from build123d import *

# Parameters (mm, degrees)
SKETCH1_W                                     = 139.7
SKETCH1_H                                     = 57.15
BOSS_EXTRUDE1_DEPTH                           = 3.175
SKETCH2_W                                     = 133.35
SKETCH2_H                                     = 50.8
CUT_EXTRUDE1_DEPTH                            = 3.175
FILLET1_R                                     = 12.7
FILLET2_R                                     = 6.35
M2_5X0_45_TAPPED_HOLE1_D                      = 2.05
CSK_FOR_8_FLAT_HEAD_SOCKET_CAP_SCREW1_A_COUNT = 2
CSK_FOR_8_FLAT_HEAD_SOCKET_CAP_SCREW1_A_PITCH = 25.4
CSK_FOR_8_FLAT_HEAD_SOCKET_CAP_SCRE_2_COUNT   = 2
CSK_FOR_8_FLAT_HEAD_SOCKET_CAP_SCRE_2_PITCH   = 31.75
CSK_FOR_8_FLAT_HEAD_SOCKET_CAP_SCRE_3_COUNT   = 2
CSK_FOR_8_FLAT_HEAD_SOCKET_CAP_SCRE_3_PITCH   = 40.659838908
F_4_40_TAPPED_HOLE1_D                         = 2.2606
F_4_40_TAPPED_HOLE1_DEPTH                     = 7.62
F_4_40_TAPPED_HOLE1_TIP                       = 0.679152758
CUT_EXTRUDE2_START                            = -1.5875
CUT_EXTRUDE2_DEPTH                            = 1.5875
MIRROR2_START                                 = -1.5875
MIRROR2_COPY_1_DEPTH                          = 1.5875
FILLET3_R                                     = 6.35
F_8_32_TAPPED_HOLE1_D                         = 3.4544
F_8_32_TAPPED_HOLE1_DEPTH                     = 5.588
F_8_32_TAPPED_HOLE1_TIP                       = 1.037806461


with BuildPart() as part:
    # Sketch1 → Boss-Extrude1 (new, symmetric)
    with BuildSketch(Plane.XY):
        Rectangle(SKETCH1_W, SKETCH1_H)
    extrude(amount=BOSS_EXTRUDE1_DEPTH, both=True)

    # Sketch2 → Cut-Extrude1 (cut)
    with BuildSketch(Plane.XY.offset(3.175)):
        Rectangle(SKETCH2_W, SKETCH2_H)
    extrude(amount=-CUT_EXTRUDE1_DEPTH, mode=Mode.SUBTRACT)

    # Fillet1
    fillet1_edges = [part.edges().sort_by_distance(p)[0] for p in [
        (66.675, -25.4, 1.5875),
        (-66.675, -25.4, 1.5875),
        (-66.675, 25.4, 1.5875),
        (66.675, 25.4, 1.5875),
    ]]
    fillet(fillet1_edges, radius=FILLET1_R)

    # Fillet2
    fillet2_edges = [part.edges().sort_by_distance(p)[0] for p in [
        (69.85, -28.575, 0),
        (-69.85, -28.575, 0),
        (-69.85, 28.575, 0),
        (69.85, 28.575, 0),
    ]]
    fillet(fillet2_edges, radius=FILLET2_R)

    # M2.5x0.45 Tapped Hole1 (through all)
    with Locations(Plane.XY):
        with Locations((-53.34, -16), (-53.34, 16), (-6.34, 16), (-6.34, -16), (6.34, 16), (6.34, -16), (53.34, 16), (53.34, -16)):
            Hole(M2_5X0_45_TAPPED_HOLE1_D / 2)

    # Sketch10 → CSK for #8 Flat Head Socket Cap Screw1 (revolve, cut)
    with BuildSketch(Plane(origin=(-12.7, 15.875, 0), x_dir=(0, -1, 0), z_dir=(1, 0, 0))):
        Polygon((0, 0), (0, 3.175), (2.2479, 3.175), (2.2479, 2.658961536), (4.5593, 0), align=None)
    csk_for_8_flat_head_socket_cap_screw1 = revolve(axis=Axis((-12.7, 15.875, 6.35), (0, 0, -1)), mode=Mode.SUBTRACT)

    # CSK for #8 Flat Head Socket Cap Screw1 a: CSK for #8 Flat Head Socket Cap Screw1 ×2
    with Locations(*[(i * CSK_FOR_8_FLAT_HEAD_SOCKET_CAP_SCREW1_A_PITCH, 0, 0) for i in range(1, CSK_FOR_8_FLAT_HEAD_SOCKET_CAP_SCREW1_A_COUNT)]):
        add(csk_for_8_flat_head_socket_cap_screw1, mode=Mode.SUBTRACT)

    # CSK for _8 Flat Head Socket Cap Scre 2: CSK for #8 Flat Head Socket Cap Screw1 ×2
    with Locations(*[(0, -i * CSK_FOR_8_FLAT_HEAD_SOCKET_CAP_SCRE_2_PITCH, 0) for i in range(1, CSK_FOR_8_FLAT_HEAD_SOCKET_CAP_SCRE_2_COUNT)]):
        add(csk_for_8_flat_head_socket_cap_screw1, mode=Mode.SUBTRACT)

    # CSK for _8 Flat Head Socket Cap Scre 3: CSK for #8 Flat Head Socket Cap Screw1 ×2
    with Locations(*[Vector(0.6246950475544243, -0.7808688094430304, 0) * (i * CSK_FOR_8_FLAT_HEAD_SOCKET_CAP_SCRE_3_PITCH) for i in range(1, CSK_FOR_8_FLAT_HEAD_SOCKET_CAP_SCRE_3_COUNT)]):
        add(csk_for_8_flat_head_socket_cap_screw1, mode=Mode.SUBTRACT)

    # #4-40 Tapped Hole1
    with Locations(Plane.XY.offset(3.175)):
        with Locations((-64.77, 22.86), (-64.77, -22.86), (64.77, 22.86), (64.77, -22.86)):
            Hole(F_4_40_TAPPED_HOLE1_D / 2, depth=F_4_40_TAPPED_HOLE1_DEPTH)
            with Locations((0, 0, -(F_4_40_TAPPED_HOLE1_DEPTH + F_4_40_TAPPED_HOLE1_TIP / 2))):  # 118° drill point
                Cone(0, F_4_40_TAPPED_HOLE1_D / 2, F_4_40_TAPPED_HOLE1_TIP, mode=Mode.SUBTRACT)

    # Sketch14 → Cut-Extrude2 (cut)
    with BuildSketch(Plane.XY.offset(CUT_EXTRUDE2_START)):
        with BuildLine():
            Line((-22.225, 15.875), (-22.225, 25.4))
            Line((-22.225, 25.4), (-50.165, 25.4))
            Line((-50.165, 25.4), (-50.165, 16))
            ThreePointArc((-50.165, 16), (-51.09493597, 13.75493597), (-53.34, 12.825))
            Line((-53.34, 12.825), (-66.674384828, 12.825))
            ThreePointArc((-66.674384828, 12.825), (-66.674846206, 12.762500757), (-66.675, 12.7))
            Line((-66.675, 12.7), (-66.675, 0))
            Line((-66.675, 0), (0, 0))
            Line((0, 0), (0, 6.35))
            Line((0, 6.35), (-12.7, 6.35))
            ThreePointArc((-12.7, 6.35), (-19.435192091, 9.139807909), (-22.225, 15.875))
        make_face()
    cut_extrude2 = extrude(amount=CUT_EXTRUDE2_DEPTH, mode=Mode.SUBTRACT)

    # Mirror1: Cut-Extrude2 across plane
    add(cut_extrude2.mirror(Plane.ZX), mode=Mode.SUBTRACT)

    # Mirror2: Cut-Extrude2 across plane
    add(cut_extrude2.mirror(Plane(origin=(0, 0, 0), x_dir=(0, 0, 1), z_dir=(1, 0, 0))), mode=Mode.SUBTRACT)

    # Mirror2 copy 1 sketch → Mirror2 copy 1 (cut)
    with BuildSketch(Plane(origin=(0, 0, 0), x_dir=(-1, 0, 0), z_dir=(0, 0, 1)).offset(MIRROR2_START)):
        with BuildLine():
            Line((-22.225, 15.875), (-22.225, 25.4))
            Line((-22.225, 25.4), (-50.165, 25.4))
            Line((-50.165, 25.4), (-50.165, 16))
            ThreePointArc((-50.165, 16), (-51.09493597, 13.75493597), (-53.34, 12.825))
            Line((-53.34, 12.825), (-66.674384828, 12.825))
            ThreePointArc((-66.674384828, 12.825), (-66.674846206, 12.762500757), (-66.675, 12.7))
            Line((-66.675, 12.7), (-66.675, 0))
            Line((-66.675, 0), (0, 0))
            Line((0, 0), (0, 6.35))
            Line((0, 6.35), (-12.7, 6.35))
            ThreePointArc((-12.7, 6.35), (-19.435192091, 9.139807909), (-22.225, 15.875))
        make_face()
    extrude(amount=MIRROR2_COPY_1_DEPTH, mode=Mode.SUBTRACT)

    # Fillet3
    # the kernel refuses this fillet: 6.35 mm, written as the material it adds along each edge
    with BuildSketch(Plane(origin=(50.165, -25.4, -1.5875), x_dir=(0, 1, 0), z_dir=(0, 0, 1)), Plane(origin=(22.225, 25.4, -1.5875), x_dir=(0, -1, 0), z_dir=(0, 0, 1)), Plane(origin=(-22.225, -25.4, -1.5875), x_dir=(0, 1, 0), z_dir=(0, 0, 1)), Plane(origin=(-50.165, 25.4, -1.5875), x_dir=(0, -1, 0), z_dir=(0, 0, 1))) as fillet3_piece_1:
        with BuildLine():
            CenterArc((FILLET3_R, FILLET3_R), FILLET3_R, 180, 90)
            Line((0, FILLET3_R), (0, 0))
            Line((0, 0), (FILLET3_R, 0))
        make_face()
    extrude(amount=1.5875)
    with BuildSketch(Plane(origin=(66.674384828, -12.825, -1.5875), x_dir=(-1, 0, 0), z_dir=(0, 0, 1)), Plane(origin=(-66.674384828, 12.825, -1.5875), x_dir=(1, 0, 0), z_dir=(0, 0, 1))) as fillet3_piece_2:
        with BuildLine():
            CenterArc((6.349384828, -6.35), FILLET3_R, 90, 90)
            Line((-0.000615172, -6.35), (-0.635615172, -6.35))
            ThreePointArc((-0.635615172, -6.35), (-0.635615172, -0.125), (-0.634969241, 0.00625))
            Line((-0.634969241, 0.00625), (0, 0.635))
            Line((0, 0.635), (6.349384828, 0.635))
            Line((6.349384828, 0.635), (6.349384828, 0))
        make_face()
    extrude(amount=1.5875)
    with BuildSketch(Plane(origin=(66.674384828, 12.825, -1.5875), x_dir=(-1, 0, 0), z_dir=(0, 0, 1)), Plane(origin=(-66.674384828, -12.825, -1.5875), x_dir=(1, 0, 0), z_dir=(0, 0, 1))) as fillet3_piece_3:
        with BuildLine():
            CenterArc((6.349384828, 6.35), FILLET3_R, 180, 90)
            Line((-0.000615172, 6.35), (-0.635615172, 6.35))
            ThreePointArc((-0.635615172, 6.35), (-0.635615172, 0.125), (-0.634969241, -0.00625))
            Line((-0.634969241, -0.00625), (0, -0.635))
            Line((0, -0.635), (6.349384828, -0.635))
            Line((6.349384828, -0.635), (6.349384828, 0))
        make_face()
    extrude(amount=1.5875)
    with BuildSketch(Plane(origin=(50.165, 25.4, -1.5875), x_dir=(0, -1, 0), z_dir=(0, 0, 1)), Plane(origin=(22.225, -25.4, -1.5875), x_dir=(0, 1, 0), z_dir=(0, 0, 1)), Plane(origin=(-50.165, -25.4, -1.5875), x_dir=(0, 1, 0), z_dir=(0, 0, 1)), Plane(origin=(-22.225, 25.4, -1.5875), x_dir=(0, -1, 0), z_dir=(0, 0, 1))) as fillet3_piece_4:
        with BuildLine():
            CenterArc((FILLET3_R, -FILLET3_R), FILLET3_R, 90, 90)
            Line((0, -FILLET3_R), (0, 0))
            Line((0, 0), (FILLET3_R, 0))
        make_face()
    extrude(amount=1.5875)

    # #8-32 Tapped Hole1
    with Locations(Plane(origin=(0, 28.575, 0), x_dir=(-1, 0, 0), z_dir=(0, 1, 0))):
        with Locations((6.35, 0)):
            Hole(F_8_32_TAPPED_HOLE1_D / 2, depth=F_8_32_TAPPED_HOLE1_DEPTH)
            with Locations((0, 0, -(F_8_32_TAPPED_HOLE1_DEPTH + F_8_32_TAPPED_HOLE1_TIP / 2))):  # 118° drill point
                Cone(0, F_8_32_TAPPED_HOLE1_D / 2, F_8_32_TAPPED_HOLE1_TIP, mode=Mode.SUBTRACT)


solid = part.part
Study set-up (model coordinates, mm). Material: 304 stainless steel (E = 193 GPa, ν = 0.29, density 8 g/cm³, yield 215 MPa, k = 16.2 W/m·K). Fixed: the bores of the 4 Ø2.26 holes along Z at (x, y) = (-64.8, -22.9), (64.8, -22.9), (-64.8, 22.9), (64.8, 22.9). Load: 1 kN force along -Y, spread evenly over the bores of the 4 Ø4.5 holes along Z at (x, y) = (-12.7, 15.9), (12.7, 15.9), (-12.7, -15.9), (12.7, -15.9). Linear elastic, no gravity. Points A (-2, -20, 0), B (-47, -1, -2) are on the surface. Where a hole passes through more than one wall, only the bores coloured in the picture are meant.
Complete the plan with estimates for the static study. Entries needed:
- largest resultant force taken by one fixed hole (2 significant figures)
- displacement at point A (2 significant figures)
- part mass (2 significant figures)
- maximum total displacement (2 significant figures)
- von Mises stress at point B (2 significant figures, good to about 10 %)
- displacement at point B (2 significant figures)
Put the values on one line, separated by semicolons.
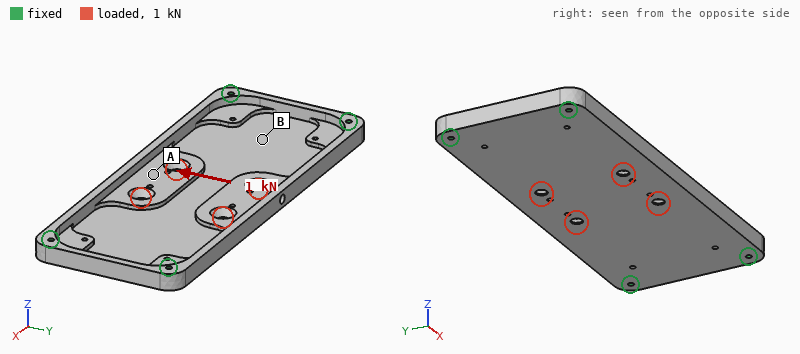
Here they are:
400 N; 7.8 µm; 180 g; 9.1 µm; 13 MPa; 1.9 µm
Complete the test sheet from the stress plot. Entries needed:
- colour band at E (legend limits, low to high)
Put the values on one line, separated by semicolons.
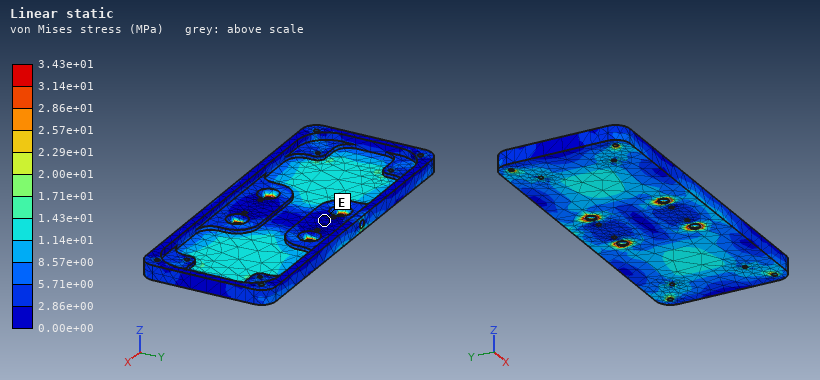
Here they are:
0.00e+00 to 2.86e+00 MPa
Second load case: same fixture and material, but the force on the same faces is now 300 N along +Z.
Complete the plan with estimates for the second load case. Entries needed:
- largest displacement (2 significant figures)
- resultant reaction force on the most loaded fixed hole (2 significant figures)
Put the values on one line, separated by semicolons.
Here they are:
88 µm; 110 N
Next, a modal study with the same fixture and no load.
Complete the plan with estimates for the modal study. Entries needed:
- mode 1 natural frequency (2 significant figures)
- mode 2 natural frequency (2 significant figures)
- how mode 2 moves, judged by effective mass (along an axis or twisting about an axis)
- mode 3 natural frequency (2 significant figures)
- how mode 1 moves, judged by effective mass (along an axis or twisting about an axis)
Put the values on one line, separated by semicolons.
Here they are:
1200 Hz; 1900 Hz; twisting about X; 3200 Hz; along Z
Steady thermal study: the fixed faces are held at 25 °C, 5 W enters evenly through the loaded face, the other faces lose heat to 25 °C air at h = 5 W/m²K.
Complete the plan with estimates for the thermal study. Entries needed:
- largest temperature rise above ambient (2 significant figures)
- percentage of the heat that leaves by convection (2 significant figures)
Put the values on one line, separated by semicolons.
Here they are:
52 K; 44 %
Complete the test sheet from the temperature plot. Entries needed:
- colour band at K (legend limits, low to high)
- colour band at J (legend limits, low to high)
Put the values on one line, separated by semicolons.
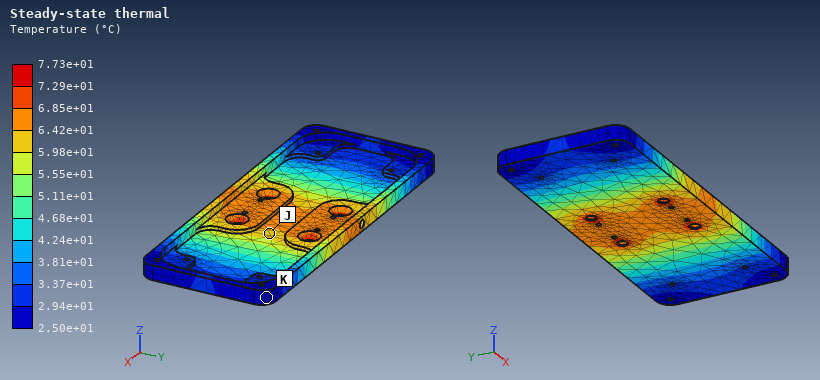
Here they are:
2.50e+01 to 2.94e+01 °C; 5.98e+01 to 6.42e+01 °C
